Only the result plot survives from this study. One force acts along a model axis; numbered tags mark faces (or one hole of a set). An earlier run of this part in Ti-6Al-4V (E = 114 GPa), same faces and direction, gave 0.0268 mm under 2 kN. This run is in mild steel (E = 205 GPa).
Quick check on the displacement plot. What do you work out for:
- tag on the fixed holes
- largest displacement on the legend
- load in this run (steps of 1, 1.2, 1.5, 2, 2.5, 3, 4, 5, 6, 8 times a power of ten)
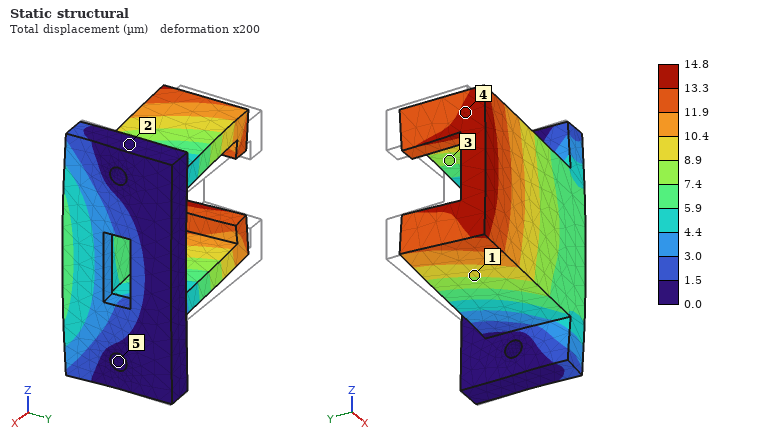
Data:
5
14.8 µm
2 kN
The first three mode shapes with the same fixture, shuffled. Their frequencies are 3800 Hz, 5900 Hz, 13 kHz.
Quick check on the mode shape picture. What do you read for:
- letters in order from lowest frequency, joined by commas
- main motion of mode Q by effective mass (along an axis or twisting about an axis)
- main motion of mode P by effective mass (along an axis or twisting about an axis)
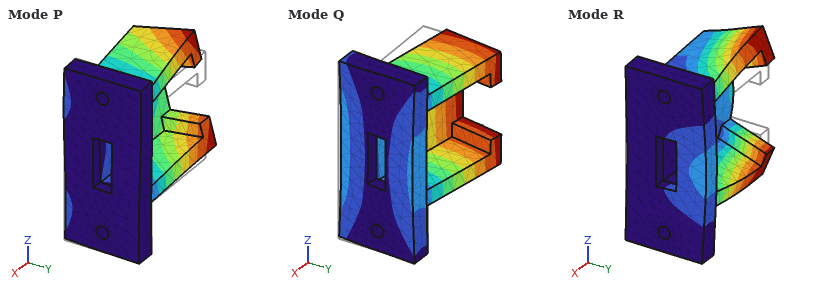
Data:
Q, P, R
along Y
along Z
